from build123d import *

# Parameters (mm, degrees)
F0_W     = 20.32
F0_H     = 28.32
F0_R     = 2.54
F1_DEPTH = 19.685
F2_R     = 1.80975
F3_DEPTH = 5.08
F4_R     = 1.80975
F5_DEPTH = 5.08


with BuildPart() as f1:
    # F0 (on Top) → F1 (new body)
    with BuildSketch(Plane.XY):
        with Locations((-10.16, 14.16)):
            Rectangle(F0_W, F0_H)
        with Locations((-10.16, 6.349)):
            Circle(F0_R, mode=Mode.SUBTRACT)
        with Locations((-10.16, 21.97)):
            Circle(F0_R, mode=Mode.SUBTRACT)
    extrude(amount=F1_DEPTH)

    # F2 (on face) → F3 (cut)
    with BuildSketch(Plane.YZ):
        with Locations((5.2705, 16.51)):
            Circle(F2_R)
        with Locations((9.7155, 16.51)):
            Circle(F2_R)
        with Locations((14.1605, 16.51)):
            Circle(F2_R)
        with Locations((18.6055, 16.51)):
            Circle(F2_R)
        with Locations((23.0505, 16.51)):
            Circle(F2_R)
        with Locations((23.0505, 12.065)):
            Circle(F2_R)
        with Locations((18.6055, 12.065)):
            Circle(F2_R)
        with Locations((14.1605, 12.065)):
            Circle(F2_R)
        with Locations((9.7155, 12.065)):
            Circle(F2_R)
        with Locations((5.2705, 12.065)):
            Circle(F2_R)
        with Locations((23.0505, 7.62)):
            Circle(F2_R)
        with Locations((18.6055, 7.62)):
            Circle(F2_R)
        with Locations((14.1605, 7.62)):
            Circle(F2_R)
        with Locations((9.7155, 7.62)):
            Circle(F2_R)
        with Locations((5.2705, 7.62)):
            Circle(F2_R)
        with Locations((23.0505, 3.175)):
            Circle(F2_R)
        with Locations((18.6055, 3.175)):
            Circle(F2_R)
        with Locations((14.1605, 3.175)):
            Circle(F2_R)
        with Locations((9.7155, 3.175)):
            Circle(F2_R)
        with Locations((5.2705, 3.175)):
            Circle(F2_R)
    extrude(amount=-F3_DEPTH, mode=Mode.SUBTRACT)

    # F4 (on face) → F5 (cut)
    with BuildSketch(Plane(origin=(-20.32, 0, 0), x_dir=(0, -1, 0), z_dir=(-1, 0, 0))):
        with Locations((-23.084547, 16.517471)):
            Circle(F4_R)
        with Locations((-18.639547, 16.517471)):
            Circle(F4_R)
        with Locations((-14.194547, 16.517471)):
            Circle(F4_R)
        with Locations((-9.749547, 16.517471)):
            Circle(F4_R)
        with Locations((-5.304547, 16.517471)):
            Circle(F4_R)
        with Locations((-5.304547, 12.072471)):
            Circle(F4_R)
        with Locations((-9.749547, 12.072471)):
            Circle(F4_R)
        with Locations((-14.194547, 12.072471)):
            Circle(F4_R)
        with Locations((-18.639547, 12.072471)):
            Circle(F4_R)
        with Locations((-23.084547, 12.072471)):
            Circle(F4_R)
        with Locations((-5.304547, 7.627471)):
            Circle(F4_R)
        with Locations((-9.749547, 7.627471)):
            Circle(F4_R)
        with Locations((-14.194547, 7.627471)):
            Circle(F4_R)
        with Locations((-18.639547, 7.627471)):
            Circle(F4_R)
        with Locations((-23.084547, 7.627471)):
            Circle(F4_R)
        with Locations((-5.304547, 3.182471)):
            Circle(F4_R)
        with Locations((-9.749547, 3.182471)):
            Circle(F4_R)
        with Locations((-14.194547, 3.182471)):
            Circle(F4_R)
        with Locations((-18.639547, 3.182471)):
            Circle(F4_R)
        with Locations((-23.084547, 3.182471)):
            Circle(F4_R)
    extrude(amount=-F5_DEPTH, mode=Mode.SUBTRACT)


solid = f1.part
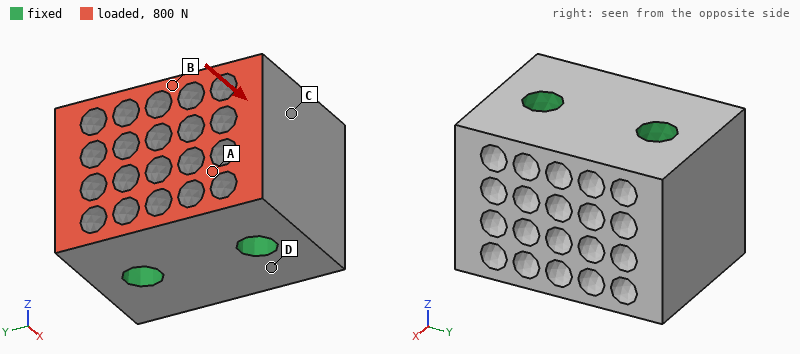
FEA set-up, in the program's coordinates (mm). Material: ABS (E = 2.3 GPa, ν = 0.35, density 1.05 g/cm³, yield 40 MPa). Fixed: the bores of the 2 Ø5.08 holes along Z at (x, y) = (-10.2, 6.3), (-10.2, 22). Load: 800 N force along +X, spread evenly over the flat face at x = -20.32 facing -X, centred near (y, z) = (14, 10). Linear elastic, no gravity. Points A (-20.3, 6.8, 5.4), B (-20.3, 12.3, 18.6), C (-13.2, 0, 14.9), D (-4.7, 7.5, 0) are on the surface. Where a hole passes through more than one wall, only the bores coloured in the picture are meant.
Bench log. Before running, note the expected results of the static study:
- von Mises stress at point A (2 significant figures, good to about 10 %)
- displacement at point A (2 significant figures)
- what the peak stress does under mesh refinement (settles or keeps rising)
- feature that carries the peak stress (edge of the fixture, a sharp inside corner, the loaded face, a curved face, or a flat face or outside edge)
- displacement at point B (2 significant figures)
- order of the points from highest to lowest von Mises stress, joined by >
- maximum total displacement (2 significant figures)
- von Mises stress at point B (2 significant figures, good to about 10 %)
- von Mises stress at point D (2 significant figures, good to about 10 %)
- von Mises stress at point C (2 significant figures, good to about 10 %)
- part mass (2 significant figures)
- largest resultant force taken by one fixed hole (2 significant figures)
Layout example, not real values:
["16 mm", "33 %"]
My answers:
["2.7 MPa", "8.5 µm", "keeps rising", "edge of the fixture", "9.6 µm", "A > B > C > D", "15 µm", "2.2 MPa", "0.50 MPa", "1.6 MPa", "8.9 g", "400 N"]
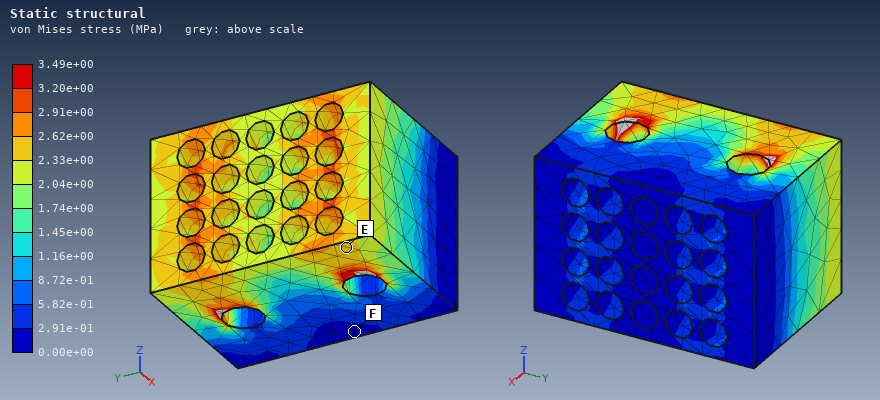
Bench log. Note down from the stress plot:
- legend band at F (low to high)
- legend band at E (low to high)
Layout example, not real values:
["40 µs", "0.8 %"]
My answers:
["0.00e+00 to 2.91e-01 MPa", "2.33e+00 to 2.62e+00 MPa"]
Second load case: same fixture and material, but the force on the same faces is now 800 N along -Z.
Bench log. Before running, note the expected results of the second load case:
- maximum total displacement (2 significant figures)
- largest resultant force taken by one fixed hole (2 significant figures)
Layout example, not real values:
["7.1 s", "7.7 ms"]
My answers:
["58 µm", "400 N"]
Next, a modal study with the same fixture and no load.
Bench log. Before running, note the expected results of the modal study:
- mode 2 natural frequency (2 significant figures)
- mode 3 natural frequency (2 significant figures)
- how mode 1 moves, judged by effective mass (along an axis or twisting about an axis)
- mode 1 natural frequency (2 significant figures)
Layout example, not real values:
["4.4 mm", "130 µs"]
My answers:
["20 kHz", "20 kHz", "twisting about Z", "18 kHz"]
